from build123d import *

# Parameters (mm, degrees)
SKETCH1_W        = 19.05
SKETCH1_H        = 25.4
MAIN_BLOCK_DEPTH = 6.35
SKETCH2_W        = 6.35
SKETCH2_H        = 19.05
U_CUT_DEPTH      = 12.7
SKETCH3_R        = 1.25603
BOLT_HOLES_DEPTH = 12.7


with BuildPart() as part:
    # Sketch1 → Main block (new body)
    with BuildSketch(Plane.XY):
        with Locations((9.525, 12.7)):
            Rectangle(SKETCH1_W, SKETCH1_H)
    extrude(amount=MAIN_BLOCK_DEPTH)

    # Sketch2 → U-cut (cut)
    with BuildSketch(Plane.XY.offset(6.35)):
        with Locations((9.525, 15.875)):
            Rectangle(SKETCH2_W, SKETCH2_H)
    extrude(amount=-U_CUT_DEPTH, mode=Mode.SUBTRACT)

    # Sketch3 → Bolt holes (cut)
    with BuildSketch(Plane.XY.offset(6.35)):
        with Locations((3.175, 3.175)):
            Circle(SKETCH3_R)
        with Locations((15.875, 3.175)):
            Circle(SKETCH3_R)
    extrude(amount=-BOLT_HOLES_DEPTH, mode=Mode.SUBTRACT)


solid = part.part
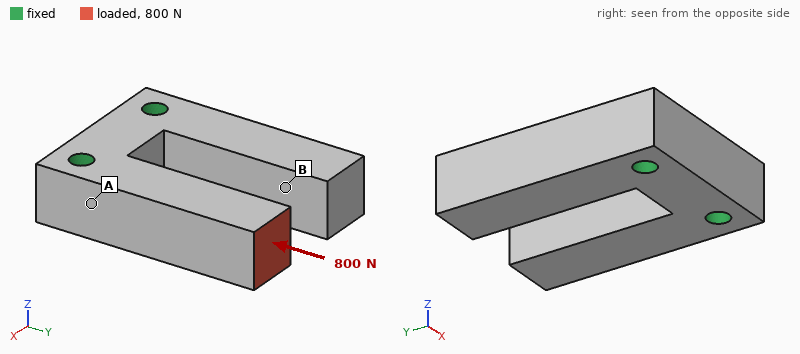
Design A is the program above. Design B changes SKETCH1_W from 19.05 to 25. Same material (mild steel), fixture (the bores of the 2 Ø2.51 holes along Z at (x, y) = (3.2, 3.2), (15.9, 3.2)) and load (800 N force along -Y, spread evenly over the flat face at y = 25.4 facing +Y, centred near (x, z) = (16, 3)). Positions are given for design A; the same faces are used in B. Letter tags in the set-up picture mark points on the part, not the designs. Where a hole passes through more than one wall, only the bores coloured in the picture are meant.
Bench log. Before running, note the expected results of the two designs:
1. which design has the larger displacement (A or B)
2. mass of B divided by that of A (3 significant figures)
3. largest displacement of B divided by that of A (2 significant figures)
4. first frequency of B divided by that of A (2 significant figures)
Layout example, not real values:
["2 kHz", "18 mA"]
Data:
["B", "1.43", "1.6", "0.99"]
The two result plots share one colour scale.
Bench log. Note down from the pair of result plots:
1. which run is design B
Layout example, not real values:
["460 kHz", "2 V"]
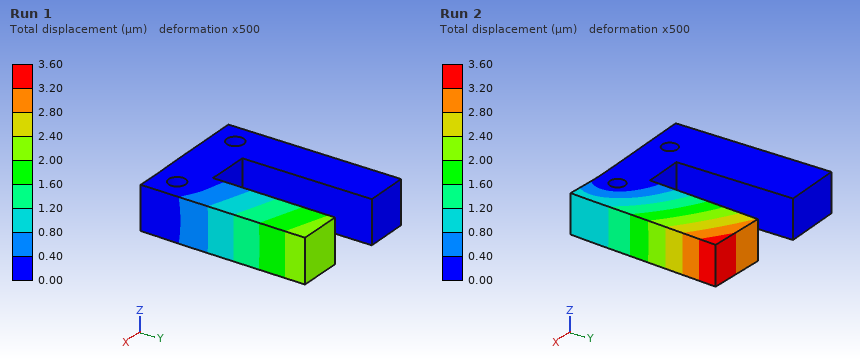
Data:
["Run 2"]
